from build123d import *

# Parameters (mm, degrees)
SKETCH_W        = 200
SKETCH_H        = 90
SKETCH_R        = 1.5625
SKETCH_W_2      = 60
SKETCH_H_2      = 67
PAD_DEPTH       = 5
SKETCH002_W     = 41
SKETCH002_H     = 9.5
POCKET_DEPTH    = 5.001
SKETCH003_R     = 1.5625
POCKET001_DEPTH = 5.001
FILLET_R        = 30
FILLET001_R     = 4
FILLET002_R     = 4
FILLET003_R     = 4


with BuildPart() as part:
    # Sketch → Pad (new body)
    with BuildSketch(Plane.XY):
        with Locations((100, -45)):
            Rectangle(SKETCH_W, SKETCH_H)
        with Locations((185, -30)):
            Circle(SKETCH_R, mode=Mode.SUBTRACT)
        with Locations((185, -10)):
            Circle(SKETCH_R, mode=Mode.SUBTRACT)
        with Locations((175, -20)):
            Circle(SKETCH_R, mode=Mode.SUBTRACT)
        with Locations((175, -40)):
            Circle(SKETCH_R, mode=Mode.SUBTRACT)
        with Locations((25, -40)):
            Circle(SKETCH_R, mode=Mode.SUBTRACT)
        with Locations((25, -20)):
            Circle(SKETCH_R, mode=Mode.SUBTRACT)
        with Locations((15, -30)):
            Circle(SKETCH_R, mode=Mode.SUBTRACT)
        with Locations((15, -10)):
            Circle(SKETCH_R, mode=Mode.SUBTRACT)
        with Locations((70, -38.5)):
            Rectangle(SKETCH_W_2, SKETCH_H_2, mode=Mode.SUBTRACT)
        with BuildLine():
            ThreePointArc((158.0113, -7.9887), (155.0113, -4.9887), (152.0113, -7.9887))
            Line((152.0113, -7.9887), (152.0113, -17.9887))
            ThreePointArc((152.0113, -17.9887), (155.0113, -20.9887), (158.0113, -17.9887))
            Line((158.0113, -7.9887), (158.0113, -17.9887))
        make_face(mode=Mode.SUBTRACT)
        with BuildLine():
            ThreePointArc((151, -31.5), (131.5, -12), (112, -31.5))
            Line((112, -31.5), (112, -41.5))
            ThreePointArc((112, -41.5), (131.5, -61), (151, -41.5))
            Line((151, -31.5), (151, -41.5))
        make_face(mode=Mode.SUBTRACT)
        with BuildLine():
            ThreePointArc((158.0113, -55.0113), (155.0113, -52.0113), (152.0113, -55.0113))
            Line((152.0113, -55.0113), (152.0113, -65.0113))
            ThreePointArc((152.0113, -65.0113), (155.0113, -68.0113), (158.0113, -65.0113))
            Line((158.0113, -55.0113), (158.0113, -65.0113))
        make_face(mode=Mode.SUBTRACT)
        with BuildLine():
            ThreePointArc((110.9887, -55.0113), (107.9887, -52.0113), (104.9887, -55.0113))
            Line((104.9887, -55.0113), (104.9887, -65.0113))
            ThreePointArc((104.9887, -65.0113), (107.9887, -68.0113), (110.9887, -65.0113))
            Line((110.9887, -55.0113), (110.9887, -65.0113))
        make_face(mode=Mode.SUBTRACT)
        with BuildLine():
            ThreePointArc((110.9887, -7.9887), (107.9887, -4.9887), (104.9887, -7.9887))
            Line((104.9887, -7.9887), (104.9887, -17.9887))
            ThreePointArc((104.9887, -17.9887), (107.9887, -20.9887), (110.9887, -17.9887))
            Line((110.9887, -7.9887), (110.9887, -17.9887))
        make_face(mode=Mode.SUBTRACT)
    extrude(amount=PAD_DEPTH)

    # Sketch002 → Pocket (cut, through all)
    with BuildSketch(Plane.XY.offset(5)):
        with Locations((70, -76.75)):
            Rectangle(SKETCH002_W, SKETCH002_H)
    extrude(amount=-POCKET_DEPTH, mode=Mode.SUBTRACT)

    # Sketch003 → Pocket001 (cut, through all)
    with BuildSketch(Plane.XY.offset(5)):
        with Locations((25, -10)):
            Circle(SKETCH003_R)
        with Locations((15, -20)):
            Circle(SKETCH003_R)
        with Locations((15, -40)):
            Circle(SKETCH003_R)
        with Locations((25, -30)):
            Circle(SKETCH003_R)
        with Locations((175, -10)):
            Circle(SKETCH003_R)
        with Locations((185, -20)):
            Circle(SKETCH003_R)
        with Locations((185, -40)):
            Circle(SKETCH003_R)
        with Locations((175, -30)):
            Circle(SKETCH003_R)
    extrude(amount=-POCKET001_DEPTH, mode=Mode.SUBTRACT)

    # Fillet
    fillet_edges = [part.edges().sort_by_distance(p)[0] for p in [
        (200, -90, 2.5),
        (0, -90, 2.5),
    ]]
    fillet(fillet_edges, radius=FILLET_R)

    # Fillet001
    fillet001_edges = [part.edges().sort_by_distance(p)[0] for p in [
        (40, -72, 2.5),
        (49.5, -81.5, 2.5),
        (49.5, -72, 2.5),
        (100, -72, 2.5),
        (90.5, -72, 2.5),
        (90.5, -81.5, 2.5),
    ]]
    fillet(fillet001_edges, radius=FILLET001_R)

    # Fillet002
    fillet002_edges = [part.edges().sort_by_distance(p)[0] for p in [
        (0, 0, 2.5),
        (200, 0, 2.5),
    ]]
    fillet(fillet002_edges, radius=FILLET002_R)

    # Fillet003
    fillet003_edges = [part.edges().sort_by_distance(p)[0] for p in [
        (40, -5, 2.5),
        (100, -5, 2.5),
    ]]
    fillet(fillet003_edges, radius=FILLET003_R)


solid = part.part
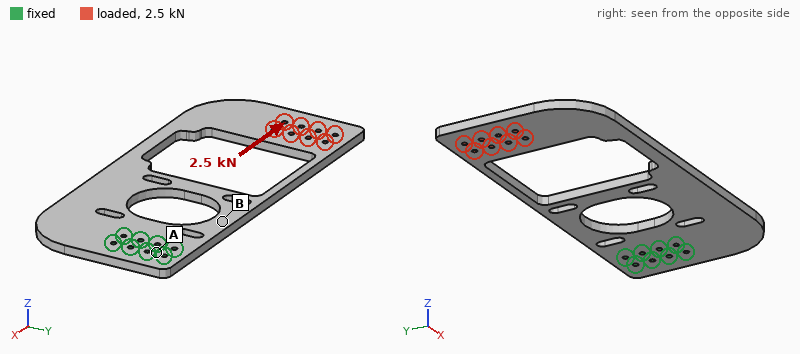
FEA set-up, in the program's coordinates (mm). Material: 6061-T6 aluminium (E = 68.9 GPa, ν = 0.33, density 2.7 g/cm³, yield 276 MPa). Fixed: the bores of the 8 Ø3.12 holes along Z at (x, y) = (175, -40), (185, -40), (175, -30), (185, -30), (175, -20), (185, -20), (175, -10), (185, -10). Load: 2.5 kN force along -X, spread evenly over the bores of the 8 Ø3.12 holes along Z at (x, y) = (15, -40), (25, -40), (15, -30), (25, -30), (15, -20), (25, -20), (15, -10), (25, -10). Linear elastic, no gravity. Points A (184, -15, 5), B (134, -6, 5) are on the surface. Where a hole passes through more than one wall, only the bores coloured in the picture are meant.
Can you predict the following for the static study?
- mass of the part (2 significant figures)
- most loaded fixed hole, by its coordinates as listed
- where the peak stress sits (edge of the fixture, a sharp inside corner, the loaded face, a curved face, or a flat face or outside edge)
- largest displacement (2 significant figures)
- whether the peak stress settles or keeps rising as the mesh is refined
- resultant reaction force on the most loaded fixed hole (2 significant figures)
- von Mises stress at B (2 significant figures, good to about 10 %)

150 g
(175, -10)
a sharp inside corner
0.15 mm
keeps rising
870 N
27 MPa
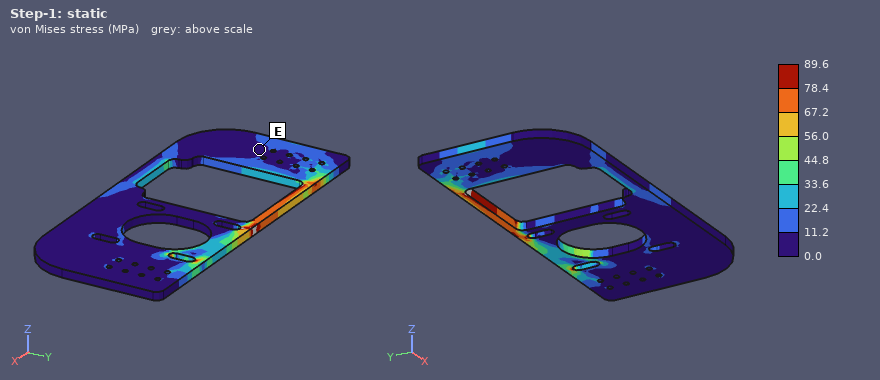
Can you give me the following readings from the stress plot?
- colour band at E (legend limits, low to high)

0.0 to 11.2 MPa
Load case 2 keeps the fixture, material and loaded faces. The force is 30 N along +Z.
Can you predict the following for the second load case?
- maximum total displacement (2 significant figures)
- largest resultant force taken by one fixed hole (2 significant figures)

2.1 mm
140 N
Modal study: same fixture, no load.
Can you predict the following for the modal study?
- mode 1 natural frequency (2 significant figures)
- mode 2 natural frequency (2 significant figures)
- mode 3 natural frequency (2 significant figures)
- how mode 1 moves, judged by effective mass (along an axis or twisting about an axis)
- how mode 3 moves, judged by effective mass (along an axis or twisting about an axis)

99 Hz
370 Hz
650 Hz
along Z
along Z
